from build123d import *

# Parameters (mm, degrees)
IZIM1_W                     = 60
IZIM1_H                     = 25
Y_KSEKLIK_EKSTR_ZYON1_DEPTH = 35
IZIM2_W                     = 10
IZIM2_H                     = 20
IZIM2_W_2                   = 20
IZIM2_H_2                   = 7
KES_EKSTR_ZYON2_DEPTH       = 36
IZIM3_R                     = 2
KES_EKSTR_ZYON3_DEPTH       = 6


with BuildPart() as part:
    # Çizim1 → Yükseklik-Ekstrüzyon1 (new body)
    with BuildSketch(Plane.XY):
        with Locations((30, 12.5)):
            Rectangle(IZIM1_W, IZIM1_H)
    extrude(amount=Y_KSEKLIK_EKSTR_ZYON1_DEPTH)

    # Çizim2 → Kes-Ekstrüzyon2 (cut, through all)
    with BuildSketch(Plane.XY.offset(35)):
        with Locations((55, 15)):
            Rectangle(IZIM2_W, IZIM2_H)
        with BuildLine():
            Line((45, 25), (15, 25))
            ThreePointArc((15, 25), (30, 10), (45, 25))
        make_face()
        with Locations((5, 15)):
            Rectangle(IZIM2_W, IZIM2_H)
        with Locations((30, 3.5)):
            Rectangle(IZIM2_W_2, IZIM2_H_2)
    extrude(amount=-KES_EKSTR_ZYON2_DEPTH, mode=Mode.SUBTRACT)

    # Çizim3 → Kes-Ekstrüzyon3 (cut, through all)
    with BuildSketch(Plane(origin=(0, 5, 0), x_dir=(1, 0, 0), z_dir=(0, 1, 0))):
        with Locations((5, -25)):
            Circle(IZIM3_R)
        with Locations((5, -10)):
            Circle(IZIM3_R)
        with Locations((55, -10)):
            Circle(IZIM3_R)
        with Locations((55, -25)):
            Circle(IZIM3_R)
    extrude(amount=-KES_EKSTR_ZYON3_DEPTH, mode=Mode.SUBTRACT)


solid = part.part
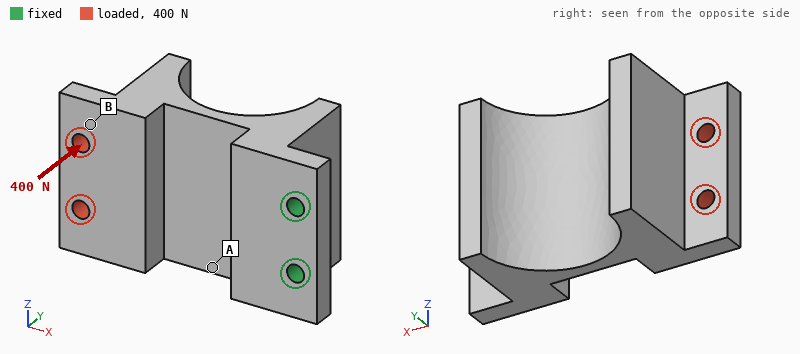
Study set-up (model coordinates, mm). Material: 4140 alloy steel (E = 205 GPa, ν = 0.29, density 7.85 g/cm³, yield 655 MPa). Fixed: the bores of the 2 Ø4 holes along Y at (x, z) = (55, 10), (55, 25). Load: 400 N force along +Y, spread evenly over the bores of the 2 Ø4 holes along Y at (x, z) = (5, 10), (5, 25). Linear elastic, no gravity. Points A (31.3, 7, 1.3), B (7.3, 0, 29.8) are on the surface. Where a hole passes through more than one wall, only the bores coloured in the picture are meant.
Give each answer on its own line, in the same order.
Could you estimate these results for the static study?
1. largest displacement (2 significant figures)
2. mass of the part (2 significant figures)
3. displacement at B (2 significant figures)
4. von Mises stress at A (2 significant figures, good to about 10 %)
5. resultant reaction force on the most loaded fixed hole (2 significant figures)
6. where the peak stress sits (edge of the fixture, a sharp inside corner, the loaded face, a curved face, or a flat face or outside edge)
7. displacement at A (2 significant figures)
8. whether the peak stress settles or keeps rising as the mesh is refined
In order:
0.32 mm
160 g
0.25 mm
180 MPa
200 N
edge of the fixture
0.050 mm
keeps rising
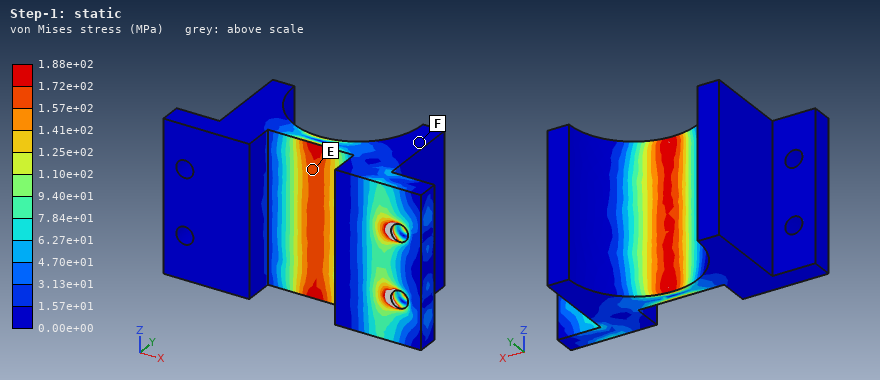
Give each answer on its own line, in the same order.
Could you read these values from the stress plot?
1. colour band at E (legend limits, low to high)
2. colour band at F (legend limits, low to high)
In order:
1.57e+02 to 1.72e+02 MPa
0.00e+00 to 1.57e+01 MPa
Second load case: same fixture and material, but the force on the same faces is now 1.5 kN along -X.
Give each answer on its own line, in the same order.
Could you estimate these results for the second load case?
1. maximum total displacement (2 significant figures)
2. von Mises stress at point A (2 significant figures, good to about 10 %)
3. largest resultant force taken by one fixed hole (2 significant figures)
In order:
0.20 mm
170 MPa
750 N
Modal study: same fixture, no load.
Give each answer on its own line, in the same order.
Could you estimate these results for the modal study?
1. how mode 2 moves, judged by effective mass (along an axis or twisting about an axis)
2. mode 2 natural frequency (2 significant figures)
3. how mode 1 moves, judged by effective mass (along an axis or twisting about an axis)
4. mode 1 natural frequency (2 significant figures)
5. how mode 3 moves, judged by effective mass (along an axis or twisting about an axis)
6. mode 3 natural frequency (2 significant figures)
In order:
twisting about X
3500 Hz
along Y
890 Hz
along Z
3900 Hz
